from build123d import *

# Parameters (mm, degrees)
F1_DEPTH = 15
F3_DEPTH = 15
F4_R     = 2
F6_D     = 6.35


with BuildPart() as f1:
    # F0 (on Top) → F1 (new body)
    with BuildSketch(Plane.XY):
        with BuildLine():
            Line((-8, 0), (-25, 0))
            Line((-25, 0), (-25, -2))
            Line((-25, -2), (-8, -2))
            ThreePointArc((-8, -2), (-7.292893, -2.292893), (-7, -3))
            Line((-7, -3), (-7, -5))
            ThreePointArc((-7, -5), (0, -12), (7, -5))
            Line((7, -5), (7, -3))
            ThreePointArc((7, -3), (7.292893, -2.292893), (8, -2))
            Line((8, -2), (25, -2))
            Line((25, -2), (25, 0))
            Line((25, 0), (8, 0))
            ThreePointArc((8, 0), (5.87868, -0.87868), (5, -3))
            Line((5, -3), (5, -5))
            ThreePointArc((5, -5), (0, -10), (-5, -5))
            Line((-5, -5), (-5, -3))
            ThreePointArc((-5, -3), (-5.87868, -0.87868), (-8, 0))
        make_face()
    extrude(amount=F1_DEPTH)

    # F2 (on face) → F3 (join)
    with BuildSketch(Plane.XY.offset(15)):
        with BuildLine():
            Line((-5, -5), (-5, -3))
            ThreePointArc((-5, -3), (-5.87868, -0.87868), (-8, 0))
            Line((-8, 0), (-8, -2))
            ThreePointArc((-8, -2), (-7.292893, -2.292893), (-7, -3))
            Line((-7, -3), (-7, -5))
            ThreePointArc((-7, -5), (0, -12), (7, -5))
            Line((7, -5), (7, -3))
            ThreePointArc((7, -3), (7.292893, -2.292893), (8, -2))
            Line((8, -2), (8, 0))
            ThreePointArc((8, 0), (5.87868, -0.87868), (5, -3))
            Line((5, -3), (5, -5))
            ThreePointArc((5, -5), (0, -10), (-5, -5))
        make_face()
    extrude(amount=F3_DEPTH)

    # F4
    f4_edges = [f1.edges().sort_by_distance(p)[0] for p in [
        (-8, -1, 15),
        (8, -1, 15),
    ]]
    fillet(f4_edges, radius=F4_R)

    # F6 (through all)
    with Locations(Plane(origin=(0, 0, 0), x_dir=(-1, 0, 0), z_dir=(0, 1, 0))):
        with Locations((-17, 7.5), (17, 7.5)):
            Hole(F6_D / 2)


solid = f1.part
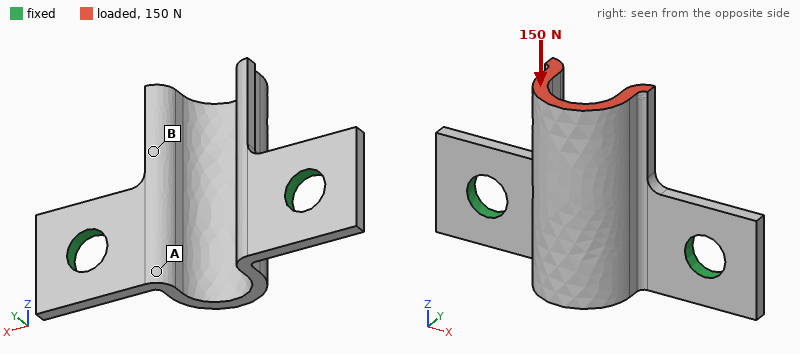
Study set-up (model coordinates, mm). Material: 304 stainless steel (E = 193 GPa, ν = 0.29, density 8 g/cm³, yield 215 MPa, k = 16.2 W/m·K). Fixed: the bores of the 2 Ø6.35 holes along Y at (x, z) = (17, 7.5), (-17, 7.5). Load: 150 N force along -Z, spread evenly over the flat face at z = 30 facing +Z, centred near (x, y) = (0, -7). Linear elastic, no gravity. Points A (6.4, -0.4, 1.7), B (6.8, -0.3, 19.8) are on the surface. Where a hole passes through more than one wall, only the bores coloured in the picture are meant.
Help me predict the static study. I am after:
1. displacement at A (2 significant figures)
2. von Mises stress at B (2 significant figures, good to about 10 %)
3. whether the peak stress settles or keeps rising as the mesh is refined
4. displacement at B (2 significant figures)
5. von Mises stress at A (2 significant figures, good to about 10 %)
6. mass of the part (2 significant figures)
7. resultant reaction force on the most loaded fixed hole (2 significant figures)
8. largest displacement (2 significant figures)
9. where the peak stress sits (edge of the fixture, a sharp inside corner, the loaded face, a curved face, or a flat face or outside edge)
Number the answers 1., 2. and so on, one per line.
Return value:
1. 4.5 µm
2. 5.1 MPa
3. keeps rising
4. 9.1 µm
5. 14 MPa
6. 21 g
7. 75 N
8. 20 µm
9. edge of the fixture
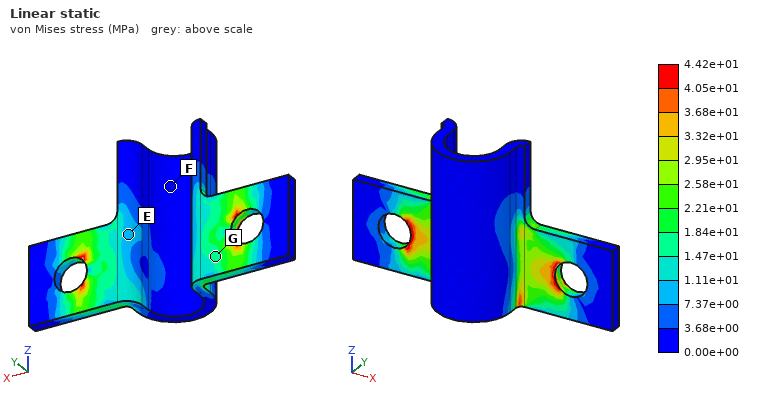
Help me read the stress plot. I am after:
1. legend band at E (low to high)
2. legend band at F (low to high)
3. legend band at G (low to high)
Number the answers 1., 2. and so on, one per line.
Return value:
1. 7.37e+00 to 1.11e+01 MPa
2. 0.00e+00 to 3.68e+00 MPa
3. 1.47e+01 to 1.84e+01 MPa
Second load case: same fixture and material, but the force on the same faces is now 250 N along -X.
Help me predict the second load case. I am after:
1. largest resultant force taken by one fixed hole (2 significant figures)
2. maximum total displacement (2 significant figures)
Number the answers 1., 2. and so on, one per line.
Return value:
1. 230 N
2. 44 µm
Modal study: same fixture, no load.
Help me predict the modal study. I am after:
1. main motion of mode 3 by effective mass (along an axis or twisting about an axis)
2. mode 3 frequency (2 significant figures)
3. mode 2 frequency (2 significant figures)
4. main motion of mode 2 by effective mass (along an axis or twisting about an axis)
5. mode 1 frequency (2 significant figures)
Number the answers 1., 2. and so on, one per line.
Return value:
1. along X
2. 11 kHz
3. 8100 Hz
4. along X
5. 3300 Hz
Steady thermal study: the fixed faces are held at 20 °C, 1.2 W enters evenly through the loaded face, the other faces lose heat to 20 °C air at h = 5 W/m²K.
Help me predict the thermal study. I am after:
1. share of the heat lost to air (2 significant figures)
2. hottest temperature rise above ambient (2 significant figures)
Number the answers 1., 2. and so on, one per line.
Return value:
1. 15 %
2. 34 K
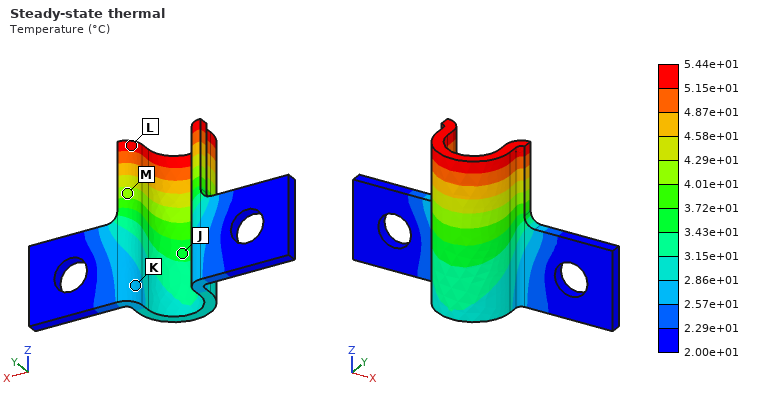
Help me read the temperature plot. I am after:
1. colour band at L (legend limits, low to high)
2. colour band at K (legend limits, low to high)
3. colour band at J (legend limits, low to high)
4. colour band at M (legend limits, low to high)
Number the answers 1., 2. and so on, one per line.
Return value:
1. 5.15e+01 to 5.44e+01 °C
2. 2.57e+01 to 2.86e+01 °C
3. 3.43e+01 to 3.72e+01 °C
4. 4.01e+01 to 4.29e+01 °C
